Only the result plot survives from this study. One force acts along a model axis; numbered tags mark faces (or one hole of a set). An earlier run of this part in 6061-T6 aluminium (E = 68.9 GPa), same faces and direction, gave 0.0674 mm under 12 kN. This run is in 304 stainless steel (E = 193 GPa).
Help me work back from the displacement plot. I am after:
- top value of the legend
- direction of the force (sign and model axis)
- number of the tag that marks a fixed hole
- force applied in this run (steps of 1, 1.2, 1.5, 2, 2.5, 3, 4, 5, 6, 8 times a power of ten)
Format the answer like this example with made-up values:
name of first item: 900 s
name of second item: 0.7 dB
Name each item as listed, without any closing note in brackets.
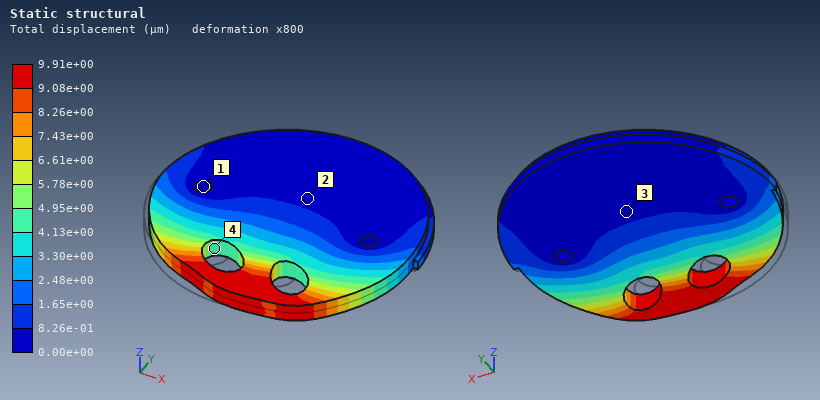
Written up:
top value of the legend: 9.91e+00 µm
direction of the force: +X
number of the tag that marks a fixed hole: 1
force applied in this run: 5 kN
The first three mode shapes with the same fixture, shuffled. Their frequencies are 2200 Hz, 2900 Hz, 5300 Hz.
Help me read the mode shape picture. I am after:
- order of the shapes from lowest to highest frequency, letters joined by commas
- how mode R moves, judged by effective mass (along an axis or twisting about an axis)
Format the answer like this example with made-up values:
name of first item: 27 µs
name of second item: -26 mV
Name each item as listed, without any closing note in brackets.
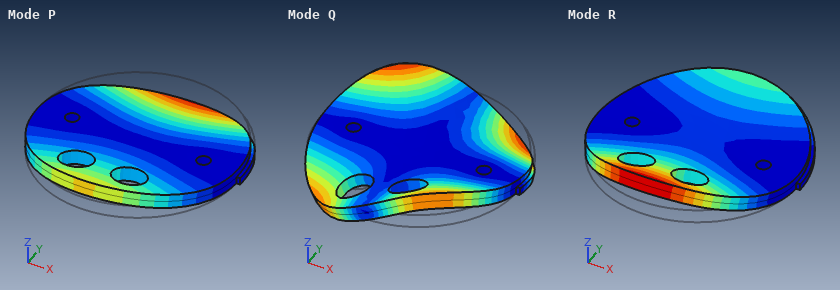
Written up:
order of the shapes from lowest to highest frequency, letters joined by commas: P, R, Q
how mode R moves, judged by effective mass: along Z
